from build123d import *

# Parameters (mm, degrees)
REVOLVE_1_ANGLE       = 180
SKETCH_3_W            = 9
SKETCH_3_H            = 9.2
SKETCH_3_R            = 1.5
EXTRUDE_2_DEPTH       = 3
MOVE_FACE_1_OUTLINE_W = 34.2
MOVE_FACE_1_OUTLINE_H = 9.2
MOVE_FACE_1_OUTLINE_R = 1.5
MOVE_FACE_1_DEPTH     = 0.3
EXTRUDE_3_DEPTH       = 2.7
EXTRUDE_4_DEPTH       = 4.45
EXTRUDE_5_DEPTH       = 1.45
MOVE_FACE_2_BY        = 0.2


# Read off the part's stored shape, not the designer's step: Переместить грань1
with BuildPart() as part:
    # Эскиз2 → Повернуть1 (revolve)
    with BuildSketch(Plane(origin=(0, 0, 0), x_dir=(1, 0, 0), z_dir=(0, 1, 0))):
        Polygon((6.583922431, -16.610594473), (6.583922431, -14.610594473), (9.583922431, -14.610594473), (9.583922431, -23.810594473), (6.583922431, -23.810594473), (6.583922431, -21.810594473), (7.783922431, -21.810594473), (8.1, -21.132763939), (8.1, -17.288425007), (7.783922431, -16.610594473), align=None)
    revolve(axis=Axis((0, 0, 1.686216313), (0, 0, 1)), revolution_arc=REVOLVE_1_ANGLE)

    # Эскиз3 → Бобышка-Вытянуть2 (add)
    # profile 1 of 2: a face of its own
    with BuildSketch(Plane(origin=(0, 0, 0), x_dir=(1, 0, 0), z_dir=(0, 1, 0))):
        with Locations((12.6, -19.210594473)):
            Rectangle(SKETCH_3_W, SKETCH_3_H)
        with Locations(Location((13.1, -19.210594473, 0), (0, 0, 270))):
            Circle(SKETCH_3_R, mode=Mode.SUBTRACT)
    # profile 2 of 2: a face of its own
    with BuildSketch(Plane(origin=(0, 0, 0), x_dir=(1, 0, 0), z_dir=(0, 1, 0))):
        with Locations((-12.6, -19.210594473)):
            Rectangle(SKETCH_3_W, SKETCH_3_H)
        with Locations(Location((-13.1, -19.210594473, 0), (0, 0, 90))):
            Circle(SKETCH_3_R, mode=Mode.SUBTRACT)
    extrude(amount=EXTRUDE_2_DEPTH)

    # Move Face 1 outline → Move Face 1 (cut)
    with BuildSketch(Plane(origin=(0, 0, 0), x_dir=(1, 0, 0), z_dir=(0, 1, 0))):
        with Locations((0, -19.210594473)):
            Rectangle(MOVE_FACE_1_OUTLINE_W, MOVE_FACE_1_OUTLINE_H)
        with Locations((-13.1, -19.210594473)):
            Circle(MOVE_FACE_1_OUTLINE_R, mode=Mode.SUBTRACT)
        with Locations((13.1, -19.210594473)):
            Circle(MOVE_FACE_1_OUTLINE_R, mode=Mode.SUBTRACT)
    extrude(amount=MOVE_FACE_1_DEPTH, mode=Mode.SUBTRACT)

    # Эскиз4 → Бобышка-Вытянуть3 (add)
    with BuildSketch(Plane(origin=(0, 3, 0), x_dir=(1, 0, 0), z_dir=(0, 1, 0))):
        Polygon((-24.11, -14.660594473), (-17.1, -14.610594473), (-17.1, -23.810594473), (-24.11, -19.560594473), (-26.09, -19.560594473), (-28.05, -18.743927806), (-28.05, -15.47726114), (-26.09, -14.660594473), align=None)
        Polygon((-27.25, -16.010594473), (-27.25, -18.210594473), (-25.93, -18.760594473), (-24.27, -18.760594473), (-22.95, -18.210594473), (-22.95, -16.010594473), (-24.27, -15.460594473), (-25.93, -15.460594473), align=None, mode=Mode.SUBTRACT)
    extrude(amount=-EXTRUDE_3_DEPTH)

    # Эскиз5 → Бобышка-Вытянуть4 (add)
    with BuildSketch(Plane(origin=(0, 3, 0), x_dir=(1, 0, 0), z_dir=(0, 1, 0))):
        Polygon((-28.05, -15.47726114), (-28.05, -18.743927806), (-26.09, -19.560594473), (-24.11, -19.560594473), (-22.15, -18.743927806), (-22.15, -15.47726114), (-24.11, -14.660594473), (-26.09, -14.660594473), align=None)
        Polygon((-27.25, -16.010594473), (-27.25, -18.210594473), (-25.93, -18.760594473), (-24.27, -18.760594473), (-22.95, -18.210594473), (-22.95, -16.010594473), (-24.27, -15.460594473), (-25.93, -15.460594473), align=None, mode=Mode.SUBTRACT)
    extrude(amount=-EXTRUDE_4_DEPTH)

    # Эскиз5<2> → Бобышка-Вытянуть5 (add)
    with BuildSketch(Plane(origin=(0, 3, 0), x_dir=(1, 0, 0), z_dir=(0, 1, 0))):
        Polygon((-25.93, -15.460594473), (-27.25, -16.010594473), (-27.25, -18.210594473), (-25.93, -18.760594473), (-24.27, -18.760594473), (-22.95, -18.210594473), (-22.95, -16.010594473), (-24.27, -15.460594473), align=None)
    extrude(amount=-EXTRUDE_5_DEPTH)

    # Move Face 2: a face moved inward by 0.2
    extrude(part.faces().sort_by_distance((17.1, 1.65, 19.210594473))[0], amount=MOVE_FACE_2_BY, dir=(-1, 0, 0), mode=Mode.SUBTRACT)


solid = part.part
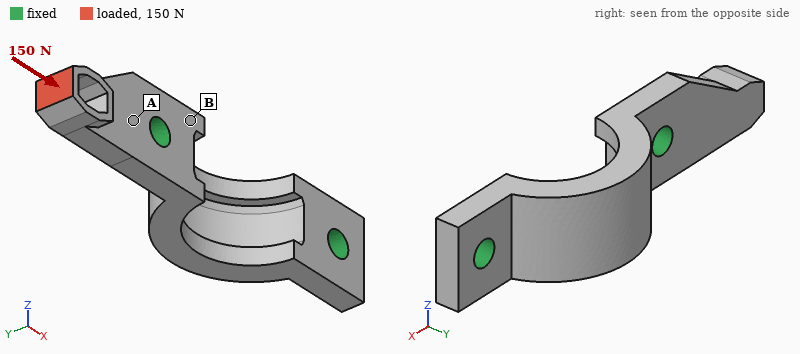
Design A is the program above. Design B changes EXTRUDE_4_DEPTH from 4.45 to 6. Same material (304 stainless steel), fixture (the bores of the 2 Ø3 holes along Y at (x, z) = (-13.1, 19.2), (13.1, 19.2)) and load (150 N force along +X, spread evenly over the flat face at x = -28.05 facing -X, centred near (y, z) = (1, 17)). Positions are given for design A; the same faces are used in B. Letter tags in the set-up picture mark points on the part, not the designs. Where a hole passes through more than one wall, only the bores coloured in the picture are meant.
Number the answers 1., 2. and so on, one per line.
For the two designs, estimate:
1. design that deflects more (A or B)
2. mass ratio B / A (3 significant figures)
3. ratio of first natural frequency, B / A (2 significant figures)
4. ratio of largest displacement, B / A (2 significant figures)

1. B
2. 1.02
3. 0.89
4. 1.7
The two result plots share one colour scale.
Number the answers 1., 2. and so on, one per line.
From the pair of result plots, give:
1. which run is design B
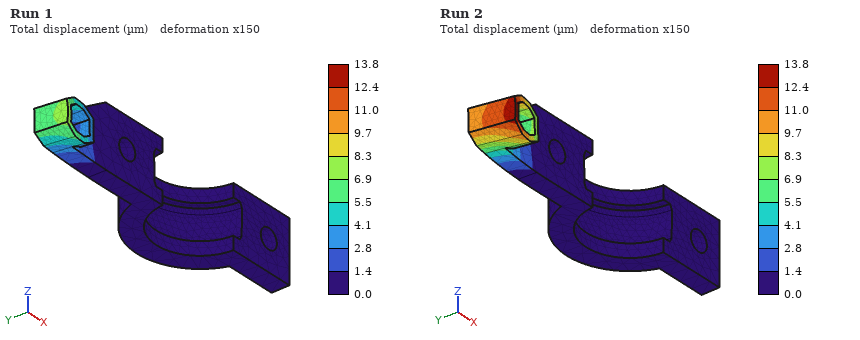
1. Run 2
